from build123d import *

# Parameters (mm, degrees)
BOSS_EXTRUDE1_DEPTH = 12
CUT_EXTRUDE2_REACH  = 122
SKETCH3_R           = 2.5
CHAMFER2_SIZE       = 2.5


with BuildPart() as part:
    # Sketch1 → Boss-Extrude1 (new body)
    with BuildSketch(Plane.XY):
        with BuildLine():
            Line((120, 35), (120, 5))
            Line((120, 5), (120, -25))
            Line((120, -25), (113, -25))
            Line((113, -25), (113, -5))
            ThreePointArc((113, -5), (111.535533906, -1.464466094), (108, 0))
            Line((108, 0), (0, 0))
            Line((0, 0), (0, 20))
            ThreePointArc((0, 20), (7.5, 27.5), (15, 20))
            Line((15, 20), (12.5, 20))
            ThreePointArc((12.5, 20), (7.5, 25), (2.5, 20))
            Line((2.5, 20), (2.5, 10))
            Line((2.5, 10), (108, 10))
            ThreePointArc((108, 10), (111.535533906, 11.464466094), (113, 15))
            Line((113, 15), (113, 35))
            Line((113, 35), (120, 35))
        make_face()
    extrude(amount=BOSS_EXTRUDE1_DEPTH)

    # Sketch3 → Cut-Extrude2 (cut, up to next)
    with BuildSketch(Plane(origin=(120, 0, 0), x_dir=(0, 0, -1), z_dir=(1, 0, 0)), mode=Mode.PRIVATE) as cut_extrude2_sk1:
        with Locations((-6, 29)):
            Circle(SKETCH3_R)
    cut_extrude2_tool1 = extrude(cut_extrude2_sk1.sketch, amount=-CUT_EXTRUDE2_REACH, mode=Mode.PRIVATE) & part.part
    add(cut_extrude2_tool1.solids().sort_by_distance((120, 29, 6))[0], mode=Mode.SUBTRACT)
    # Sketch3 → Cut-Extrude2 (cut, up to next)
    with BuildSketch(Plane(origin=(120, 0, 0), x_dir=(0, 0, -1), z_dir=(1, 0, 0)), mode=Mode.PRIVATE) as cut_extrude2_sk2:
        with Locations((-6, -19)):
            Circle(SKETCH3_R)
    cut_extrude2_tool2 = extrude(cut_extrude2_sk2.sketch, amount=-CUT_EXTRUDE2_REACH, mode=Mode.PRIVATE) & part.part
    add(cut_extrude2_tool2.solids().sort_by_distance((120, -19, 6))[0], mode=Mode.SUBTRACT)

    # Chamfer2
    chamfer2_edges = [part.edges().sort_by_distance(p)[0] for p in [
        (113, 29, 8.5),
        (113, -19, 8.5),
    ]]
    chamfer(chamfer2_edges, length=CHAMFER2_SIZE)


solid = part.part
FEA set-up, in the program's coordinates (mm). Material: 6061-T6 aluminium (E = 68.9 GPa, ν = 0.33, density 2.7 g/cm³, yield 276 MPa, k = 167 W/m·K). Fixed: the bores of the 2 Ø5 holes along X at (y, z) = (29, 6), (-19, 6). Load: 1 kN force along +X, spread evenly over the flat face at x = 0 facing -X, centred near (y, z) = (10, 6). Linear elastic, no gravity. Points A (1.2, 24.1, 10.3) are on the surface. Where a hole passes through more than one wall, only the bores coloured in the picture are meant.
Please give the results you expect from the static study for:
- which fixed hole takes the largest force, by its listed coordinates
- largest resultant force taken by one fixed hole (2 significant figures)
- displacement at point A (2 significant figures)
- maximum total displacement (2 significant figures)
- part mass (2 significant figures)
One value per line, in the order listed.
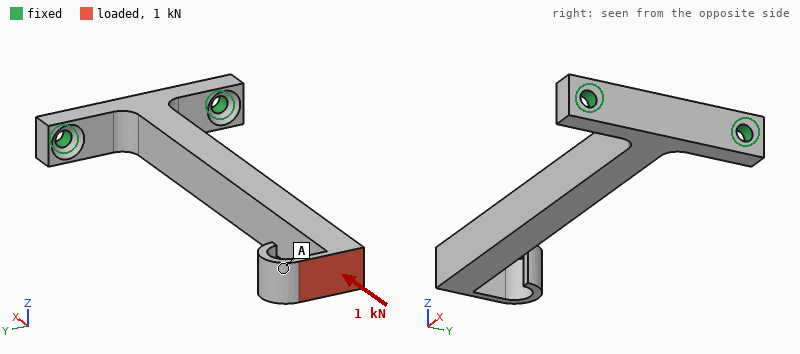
(29, 6)
760 N
0.59 mm
0.59 mm
52 g
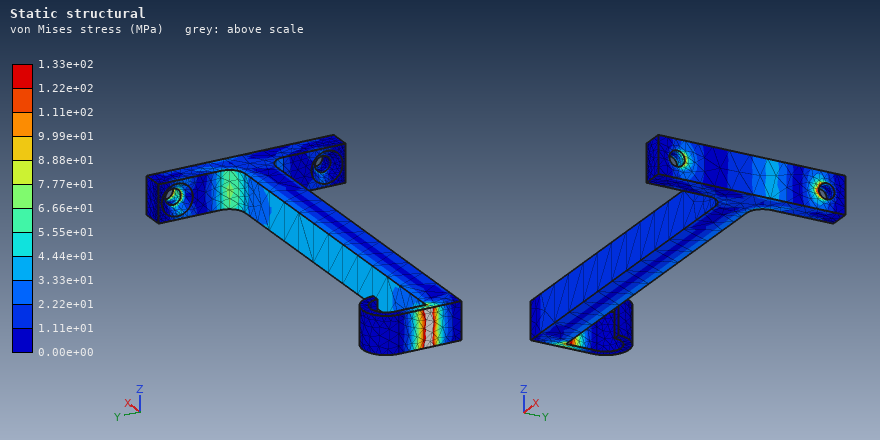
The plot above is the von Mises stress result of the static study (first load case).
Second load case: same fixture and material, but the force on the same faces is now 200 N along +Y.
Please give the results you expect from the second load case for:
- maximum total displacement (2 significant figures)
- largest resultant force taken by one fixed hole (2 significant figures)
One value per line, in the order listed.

1.6 mm
660 N
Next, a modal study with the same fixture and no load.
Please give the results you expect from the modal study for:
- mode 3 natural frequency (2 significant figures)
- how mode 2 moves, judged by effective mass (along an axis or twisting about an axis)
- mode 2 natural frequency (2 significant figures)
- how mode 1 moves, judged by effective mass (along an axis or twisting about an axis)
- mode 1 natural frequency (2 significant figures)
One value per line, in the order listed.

2700 Hz
along Y
530 Hz
along Z
420 Hz
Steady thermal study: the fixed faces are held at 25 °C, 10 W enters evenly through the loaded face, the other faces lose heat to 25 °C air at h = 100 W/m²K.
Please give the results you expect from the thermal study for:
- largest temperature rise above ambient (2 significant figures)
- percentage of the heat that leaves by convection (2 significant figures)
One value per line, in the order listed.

29 K
77 %
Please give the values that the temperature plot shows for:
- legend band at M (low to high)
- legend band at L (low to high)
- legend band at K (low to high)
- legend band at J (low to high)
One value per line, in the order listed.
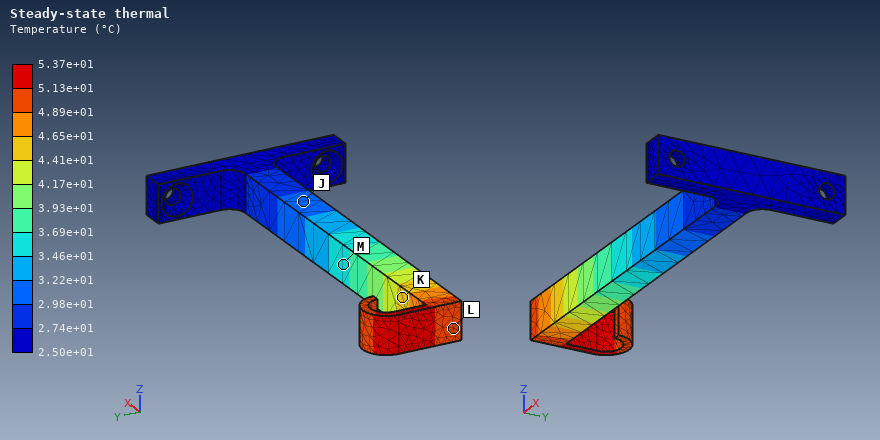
3.46e+01 to 3.69e+01 °C
4.89e+01 to 5.13e+01 °C
4.41e+01 to 4.65e+01 °C
2.98e+01 to 3.22e+01 °C
